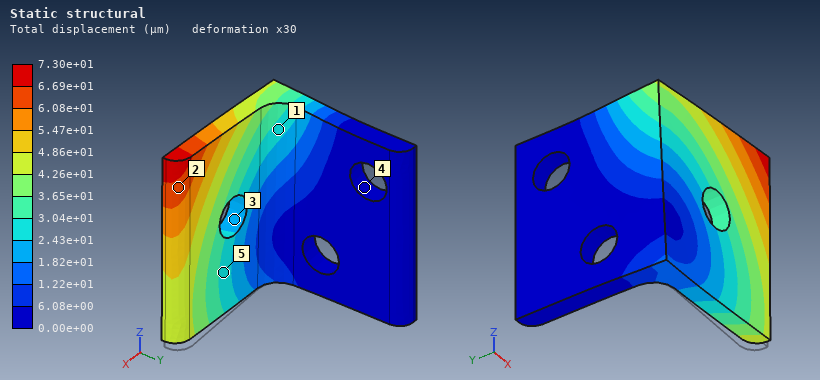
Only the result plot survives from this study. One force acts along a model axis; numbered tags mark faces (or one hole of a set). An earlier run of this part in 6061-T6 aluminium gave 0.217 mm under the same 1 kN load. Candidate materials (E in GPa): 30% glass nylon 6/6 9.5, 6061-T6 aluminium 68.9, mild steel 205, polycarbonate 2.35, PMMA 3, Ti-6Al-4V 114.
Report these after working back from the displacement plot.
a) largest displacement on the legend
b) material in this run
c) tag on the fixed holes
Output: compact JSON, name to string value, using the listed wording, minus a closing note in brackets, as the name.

{"largest displacement on the legend": "7.30e+01 µm", "material in this run": "mild steel", "tag on the fixed holes": "4"}
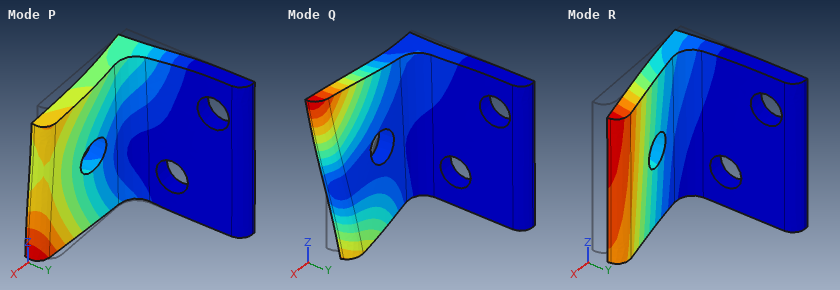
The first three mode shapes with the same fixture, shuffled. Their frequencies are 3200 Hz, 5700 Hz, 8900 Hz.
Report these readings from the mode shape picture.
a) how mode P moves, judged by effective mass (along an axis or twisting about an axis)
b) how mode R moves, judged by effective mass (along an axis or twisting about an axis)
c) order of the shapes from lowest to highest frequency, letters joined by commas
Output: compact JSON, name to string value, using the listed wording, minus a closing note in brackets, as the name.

{"how mode P moves, judged by effective mass": "along Z", "how mode R moves, judged by effective mass": "along Y", "order of the shapes from lowest to highest frequency, letters joined by commas": "R, P, Q"}
